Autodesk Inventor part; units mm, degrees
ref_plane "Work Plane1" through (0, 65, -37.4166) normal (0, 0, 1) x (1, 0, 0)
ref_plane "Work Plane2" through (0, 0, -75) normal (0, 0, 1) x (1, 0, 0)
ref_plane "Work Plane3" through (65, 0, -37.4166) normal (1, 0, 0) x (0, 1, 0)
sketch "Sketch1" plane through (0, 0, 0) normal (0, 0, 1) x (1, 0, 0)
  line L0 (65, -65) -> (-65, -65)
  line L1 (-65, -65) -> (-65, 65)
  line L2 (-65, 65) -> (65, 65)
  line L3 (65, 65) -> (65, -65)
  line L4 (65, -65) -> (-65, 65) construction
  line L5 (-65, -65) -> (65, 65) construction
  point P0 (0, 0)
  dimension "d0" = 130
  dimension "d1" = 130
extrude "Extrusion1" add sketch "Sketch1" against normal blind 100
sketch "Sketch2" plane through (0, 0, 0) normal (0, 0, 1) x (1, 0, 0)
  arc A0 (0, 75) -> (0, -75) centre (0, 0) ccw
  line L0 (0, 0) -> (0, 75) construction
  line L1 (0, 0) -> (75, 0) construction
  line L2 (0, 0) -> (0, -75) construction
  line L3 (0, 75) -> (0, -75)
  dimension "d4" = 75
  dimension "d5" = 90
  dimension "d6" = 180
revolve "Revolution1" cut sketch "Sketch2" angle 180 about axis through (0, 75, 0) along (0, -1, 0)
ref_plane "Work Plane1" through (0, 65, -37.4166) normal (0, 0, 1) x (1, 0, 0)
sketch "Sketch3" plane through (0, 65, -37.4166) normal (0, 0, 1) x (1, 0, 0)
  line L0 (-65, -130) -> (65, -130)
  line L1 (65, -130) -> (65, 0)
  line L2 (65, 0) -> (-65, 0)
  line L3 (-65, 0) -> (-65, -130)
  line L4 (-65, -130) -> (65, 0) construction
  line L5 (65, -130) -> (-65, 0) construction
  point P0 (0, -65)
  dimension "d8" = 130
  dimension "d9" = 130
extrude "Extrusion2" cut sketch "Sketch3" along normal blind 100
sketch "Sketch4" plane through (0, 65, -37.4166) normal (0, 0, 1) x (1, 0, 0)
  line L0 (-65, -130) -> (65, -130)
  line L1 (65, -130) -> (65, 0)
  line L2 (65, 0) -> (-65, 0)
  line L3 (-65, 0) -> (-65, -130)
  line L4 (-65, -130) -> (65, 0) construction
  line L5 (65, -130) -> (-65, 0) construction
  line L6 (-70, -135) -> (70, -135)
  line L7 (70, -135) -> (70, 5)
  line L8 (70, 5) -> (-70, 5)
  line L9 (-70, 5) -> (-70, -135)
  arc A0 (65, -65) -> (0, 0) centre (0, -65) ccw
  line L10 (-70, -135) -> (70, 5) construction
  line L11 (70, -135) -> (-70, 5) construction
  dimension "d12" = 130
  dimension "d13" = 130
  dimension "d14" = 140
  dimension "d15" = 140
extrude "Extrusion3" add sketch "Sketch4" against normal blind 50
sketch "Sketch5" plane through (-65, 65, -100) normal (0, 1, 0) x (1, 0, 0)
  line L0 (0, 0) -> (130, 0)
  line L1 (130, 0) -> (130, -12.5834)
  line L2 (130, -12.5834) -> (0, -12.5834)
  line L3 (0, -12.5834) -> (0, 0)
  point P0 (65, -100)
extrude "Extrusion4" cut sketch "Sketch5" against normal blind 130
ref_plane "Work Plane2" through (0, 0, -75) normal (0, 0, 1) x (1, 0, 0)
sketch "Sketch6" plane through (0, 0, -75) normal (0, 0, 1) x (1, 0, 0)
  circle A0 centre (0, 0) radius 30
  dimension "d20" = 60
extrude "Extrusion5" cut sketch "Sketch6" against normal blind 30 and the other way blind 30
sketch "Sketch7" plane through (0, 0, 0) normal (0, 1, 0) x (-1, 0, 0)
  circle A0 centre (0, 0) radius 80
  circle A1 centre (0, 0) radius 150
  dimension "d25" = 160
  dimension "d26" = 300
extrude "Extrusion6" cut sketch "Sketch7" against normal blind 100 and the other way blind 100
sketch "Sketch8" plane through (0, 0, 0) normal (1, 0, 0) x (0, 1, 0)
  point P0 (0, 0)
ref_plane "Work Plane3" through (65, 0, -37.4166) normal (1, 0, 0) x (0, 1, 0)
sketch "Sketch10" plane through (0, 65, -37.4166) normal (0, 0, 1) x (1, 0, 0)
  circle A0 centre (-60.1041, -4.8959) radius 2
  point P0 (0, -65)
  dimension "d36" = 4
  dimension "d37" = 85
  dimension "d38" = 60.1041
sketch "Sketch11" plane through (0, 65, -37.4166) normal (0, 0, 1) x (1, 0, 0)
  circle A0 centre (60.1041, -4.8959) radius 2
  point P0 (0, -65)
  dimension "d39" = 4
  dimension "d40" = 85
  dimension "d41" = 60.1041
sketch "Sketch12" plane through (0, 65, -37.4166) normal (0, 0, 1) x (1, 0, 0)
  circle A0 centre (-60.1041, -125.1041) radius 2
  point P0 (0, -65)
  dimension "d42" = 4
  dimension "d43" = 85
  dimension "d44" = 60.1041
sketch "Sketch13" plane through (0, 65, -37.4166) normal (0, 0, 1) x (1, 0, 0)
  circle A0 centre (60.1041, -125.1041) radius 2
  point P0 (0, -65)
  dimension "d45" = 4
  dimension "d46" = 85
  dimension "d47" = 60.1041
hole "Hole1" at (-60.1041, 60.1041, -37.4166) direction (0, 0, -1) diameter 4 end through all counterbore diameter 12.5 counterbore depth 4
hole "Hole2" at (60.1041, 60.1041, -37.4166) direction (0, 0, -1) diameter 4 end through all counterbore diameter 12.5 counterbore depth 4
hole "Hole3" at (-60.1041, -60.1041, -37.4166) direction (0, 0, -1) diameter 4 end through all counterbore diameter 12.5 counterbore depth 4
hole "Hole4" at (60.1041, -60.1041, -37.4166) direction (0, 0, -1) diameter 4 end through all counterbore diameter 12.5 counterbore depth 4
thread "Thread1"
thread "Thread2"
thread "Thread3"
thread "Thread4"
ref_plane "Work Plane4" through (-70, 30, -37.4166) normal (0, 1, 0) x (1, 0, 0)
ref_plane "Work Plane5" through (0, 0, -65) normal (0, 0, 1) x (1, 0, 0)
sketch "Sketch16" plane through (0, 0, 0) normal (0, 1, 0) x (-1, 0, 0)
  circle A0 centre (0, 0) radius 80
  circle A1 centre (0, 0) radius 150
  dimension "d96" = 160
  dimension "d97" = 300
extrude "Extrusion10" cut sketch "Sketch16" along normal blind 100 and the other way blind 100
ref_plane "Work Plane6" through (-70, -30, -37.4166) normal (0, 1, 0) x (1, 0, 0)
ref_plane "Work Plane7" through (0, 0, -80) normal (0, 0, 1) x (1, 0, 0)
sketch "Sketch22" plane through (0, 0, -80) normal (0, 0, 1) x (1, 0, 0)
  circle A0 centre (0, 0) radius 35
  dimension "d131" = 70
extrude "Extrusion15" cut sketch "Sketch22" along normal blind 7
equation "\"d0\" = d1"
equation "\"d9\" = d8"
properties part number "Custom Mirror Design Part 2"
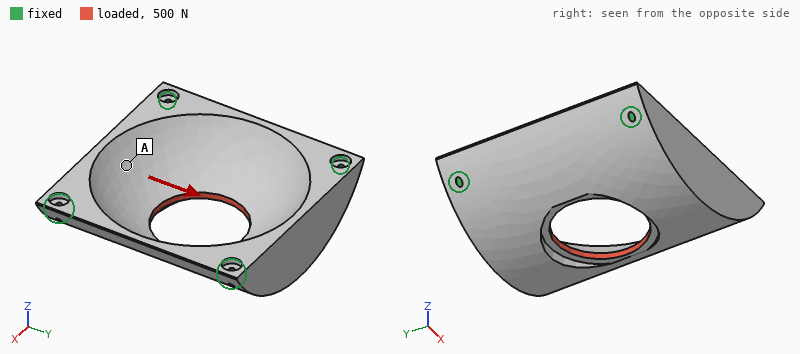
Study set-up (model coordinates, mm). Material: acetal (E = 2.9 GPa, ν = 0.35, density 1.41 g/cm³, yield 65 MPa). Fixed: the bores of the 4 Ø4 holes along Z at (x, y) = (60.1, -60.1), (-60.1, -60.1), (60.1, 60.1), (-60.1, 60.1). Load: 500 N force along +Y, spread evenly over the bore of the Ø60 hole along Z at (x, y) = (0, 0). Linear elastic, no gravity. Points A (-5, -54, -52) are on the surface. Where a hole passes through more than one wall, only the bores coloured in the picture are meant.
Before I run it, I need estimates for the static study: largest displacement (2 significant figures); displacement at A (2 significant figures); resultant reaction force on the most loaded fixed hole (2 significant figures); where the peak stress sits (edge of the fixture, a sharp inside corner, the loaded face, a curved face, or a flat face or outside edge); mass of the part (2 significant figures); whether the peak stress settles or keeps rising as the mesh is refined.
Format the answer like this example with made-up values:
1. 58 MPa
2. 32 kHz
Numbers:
1. 20 µm
2. 11 µm
3. 140 N
4. edge of the fixture
5. 420 g
6. keeps rising
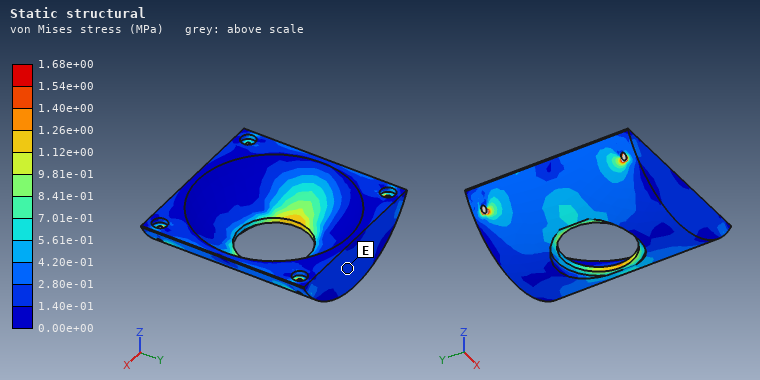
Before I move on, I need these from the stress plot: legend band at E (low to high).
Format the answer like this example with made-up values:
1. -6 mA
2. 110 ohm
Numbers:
1. 1.40e-01 to 2.80e-01 MPa
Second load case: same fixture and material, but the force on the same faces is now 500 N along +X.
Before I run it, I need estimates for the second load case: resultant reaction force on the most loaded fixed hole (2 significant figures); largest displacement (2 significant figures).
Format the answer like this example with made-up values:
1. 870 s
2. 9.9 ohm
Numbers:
1. 140 N
2. 52 µm
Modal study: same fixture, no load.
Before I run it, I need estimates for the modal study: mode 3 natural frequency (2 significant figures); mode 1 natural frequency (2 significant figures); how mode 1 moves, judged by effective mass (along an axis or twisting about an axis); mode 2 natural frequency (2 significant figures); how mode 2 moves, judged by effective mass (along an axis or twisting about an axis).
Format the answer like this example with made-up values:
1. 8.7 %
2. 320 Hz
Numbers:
1. 1500 Hz
2. 1200 Hz
3. along Z
4. 1400 Hz
5. along Z
